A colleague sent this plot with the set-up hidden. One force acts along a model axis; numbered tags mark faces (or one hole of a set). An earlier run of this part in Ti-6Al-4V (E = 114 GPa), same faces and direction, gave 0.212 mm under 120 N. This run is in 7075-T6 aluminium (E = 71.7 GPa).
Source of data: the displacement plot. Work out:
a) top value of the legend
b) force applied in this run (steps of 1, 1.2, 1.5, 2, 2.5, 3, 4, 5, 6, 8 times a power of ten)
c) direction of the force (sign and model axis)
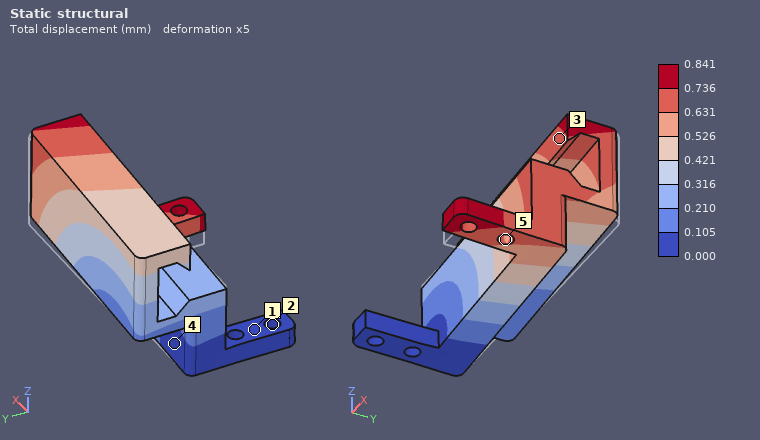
0.841 mm
300 N
+Z
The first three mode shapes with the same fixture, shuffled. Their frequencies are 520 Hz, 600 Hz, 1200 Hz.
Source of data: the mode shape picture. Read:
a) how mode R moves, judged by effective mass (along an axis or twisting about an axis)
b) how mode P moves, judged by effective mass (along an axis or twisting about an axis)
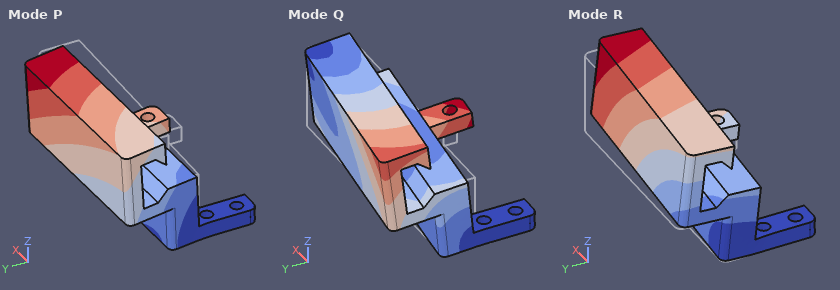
along Z
along Y
